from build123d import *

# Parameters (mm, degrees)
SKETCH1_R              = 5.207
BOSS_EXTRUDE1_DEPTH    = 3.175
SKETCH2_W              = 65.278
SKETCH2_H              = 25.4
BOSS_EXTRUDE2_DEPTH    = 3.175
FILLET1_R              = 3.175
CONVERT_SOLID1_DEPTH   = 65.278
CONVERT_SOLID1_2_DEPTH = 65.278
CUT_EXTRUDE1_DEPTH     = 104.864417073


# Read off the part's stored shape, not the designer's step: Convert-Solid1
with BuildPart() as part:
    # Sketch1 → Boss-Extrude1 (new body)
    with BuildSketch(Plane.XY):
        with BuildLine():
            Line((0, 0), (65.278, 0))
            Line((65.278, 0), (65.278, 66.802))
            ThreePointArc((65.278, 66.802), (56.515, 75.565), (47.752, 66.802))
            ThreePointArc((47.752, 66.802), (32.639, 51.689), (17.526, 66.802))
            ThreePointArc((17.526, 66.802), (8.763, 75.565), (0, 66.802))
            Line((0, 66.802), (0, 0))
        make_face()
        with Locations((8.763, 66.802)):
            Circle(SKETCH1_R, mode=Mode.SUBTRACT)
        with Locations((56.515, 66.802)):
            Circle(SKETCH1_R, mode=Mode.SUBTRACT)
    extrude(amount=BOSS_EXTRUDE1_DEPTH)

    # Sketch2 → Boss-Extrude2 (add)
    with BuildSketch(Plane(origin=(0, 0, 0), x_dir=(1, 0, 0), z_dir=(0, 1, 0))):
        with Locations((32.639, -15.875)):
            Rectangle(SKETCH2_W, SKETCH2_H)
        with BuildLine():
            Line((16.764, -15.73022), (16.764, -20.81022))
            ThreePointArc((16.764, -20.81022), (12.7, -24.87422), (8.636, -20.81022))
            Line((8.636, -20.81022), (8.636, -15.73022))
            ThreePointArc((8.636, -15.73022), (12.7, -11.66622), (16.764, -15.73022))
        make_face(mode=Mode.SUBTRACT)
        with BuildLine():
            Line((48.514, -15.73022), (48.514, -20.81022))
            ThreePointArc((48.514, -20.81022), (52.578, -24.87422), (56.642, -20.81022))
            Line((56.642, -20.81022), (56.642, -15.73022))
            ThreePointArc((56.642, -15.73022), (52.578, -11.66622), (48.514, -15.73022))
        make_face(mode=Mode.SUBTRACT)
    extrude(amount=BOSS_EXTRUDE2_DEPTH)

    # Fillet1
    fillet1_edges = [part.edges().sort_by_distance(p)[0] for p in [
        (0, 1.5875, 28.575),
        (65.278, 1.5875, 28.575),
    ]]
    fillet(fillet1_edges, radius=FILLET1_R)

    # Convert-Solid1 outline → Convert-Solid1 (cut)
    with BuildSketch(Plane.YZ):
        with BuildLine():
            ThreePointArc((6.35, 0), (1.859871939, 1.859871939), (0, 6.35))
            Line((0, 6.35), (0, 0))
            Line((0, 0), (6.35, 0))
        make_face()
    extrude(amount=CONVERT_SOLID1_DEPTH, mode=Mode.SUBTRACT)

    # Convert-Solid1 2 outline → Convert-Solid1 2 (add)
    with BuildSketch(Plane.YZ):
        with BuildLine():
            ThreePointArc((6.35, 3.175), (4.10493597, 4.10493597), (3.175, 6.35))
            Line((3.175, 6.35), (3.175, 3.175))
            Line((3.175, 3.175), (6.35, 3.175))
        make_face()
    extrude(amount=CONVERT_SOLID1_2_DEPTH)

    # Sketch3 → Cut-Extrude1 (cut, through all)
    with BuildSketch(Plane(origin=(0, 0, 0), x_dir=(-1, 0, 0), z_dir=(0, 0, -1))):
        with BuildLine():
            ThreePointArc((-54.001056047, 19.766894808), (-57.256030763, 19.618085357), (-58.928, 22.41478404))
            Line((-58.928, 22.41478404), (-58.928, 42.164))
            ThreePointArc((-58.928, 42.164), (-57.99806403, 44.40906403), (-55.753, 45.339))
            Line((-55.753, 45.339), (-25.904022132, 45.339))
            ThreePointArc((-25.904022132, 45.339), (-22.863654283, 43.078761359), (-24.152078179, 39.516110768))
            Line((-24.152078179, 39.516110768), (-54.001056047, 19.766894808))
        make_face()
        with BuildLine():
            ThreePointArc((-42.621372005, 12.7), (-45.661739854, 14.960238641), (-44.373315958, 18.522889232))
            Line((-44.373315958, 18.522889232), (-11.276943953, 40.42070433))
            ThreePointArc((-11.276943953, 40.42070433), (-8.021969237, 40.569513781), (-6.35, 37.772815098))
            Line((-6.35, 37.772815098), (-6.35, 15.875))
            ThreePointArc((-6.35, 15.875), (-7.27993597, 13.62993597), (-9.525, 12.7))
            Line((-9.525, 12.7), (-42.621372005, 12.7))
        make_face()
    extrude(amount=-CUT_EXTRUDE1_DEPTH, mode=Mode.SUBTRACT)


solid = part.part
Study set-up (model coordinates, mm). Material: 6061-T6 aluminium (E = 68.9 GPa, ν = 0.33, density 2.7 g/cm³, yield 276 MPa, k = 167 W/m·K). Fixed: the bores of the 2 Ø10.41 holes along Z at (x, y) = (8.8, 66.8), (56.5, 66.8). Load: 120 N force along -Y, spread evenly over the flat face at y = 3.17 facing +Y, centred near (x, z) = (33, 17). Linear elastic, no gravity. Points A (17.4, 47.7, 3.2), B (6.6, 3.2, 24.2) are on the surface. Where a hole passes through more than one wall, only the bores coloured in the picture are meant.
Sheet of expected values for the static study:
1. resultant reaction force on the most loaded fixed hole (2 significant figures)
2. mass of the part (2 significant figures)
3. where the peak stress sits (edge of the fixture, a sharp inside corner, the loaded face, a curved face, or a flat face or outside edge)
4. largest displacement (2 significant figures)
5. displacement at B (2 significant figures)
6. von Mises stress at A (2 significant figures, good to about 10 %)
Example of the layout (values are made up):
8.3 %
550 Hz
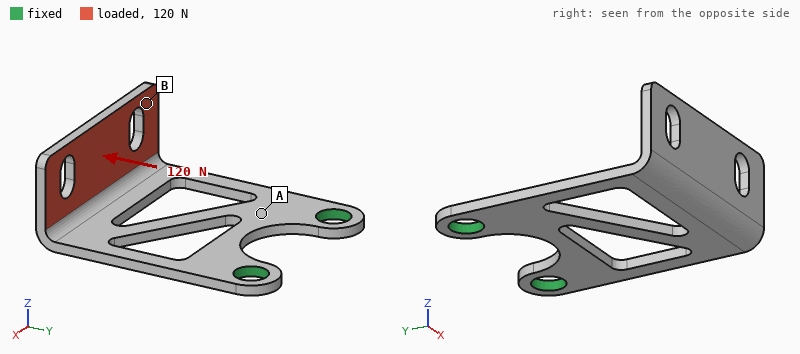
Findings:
64 N
35 g
a curved face
1.1 mm
0.95 mm
24 MPa
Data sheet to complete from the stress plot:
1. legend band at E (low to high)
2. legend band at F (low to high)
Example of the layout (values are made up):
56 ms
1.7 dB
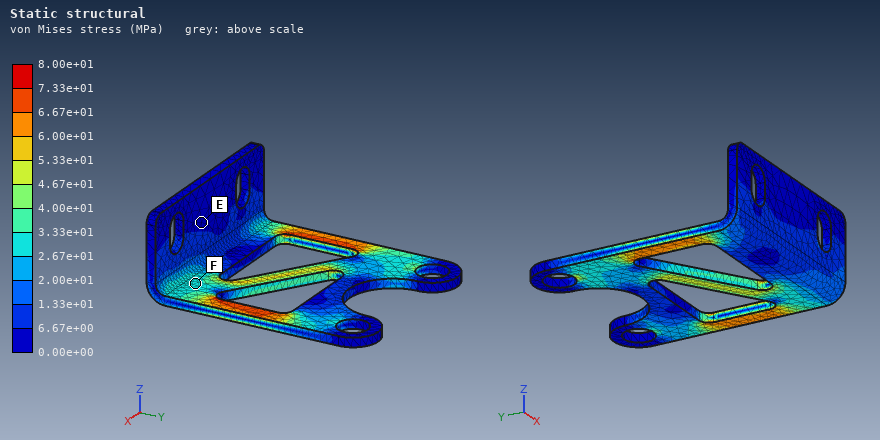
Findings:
0.00e+00 to 6.67e+00 MPa
2.67e+01 to 3.33e+01 MPa
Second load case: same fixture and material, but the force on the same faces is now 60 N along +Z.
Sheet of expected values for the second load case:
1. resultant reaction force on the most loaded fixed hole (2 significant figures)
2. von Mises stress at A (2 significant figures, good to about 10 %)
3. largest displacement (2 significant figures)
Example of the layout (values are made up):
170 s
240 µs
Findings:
31 N
32 MPa
1.1 mm
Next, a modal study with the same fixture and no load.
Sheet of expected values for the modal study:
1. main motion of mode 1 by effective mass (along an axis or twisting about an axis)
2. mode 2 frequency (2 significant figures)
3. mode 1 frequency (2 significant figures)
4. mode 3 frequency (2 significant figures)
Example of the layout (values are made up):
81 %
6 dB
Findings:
along Z
760 Hz
290 Hz
1400 Hz
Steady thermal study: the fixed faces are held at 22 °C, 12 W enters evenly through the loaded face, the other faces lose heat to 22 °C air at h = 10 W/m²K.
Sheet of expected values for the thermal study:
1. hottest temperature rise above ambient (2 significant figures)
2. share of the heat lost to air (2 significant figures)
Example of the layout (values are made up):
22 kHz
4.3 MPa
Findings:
54 K
22 %
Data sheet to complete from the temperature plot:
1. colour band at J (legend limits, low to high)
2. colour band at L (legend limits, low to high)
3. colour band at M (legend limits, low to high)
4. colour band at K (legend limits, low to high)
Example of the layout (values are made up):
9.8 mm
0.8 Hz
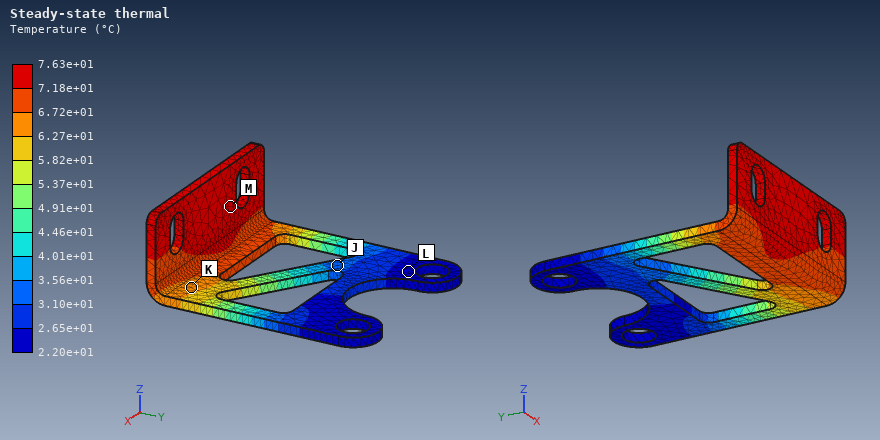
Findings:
3.10e+01 to 3.56e+01 °C
2.20e+01 to 2.65e+01 °C
7.18e+01 to 7.63e+01 °C
6.27e+01 to 6.72e+01 °C
